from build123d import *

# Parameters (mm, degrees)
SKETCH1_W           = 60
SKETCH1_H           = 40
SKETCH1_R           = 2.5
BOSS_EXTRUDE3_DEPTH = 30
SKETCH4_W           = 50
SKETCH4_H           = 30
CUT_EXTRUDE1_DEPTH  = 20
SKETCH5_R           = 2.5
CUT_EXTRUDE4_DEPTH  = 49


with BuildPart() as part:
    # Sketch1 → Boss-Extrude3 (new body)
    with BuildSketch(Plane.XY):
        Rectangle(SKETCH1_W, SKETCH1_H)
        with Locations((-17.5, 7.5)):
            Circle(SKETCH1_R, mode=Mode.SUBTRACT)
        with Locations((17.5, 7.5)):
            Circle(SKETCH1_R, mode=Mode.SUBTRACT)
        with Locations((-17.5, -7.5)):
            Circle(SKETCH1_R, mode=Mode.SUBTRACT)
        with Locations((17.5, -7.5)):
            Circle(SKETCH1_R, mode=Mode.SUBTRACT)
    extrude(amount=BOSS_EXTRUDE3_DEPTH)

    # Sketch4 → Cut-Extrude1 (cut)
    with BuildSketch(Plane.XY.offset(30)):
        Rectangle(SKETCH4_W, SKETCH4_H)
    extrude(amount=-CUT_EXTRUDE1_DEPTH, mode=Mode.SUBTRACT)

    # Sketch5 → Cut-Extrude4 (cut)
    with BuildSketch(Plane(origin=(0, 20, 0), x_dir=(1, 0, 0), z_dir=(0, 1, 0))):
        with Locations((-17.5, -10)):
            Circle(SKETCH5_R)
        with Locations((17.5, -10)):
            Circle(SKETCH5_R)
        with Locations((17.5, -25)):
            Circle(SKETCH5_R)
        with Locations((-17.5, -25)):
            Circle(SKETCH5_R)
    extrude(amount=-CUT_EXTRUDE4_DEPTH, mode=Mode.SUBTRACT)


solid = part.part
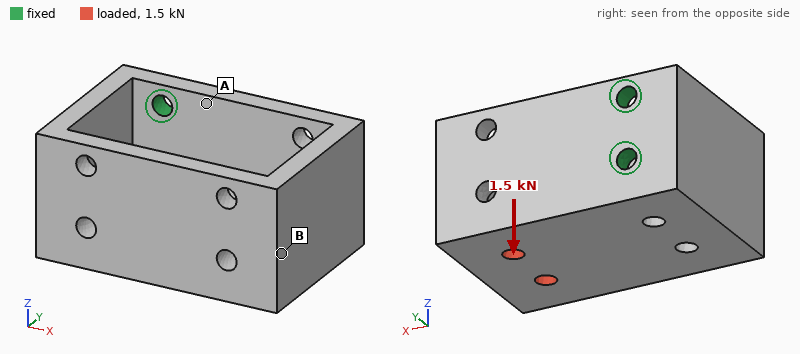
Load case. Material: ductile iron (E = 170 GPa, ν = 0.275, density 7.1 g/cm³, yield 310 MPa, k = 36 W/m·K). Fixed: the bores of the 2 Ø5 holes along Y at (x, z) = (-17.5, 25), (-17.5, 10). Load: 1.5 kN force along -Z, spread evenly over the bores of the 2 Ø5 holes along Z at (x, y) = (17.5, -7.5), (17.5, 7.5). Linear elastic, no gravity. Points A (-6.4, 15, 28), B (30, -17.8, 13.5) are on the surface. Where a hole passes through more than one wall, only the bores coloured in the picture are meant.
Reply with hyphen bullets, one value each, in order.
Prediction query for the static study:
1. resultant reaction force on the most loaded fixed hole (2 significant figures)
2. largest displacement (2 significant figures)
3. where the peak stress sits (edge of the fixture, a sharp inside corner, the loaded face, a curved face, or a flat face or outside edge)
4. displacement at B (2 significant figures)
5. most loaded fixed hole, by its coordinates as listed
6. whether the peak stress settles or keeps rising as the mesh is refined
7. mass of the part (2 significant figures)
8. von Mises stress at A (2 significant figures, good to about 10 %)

- 3.0 kN
- 68 µm
- edge of the fixture
- 59 µm
- (-17.5, 10)
- keeps rising
- 280 g
- 29 MPa
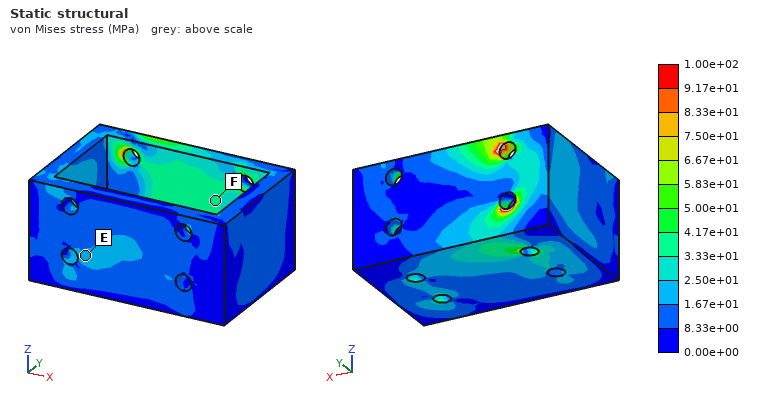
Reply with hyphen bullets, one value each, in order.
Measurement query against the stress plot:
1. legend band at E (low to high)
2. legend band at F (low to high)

- 1.67e+01 to 2.50e+01 MPa
- 3.33e+01 to 4.17e+01 MPa
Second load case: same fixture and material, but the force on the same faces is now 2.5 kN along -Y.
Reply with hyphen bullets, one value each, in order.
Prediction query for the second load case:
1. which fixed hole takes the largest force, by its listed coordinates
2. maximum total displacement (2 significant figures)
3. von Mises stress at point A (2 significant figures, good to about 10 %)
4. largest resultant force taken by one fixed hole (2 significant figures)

- (-17.5, 10)
- 88 µm
- 46 MPa
- 2.8 kN
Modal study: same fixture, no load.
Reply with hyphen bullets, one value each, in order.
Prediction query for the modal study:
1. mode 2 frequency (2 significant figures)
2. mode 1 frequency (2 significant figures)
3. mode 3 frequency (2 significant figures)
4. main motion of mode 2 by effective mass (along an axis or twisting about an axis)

- 2300 Hz
- 2200 Hz
- 5500 Hz
- along Z
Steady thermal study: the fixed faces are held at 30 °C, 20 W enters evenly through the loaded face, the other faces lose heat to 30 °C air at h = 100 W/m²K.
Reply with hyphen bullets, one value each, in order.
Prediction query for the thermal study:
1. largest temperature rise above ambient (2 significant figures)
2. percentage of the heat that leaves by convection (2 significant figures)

- 28 K
- 71 %
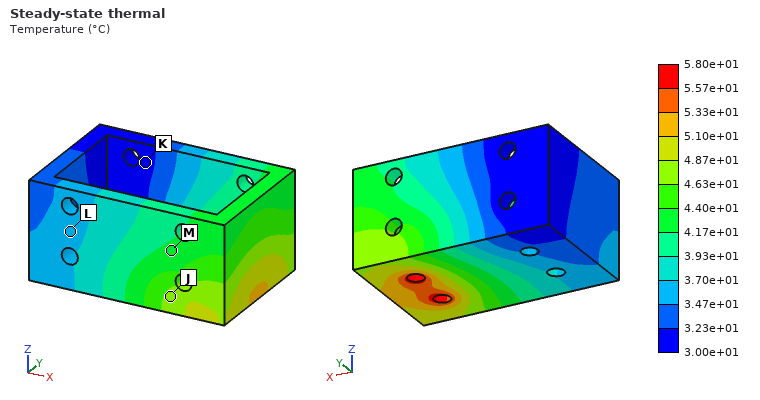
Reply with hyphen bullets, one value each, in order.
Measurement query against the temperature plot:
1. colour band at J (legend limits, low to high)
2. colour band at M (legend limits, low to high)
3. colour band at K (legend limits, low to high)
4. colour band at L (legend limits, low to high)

- 4.63e+01 to 4.87e+01 °C
- 4.17e+01 to 4.40e+01 °C
- 3.00e+01 to 3.23e+01 °C
- 3.47e+01 to 3.70e+01 °C
